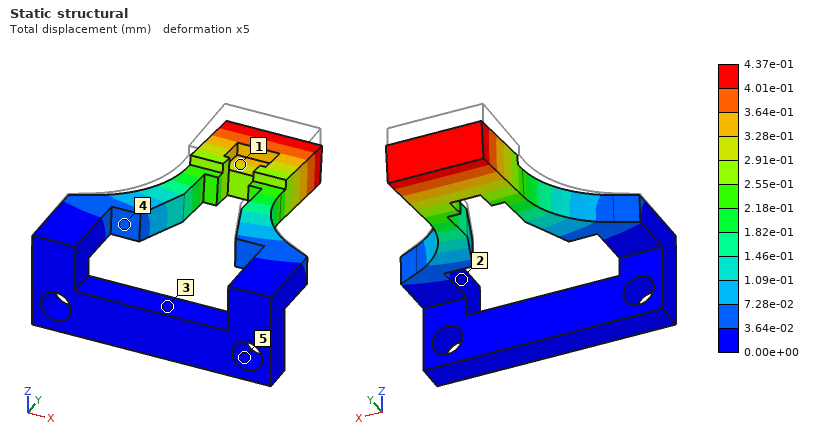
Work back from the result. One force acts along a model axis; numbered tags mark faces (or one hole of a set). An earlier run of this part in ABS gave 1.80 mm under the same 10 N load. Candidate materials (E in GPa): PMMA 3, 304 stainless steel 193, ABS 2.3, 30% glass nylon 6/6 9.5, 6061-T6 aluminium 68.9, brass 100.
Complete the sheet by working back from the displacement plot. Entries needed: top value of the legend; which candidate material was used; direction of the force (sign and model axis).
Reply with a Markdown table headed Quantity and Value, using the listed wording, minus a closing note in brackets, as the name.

| Quantity | Value |
|---|---|
| top value of the legend | 4.37e-01 mm |
| which candidate material was used | 30% glass nylon 6/6 |
| direction of the force | -Z |
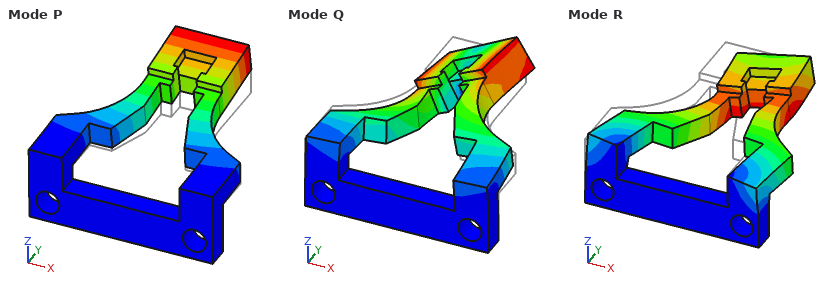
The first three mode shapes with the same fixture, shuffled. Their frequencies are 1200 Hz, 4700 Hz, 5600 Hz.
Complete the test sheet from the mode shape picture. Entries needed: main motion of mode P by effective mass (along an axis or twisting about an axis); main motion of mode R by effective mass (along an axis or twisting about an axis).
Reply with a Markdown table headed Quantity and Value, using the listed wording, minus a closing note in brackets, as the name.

| Quantity | Value |
|---|---|
| main motion of mode P by effective mass | along Z |
| main motion of mode R by effective mass | along X |
